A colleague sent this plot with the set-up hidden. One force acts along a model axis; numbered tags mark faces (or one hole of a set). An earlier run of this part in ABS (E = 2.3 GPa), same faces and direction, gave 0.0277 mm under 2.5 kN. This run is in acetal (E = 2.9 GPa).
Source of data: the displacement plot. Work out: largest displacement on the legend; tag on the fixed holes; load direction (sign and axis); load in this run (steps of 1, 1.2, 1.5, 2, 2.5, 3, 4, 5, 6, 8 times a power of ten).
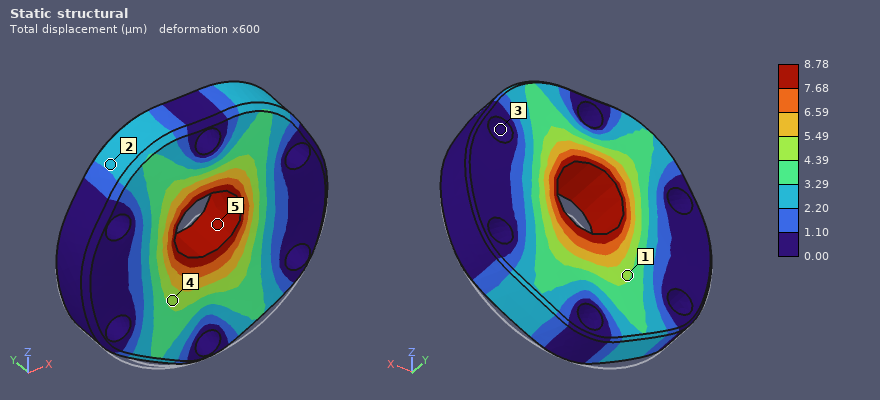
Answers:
8.78 µm
3
+Z
1 kN
